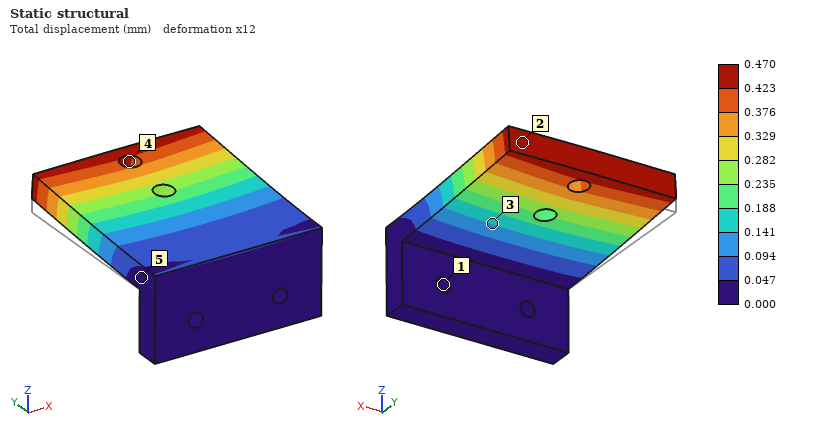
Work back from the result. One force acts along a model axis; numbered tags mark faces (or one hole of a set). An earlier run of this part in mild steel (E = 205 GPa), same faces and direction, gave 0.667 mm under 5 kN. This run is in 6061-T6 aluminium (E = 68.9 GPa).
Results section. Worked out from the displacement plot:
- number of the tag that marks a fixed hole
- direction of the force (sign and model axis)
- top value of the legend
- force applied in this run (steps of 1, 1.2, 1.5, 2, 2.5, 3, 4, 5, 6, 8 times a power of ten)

1
+Z
0.470 mm
1.2 kN
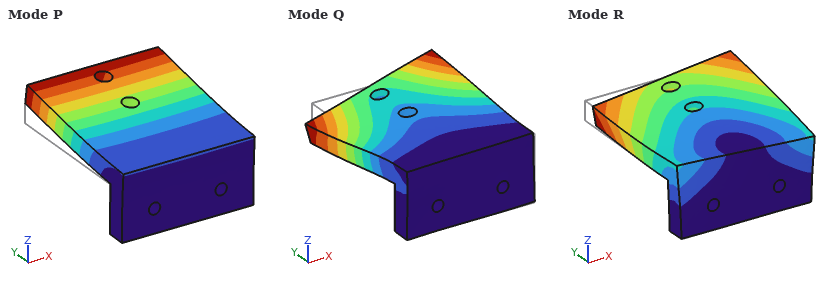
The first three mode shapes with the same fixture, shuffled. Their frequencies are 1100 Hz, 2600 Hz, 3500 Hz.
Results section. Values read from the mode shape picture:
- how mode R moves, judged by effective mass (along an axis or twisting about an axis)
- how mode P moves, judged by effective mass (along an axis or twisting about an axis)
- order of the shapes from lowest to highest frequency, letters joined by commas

along X
along Z
P, R, Q
